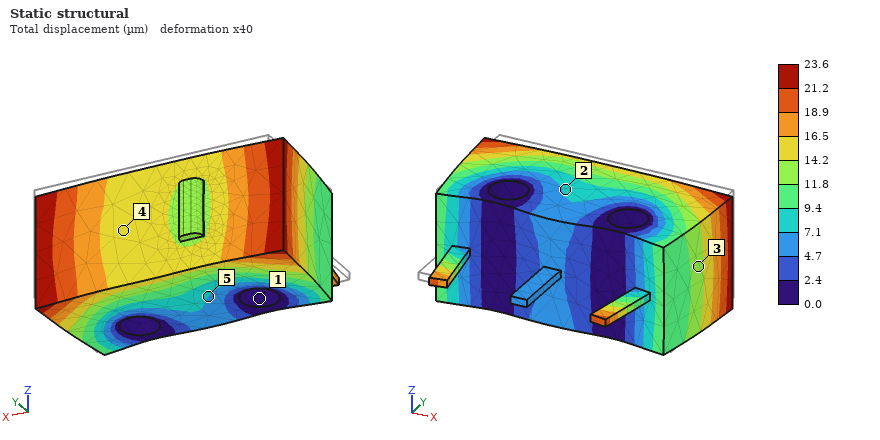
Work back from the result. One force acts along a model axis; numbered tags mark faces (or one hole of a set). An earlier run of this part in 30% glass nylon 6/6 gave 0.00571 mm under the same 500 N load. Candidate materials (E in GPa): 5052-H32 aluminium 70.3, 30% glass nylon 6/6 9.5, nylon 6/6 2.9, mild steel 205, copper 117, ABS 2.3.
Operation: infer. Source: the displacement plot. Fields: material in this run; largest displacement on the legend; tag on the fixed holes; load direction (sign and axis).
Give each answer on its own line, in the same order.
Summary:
ABS
23.6 µm
1
-Y
